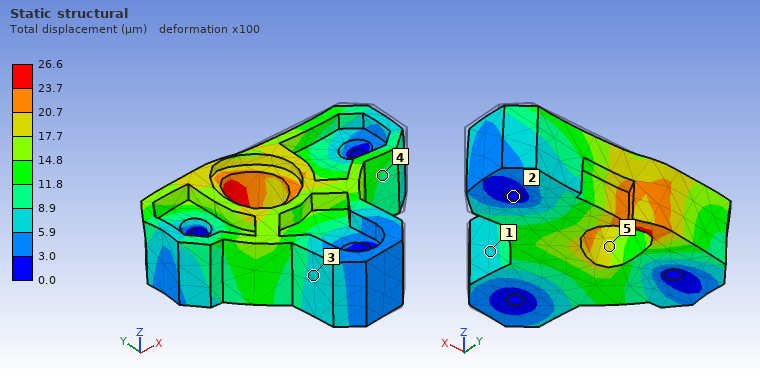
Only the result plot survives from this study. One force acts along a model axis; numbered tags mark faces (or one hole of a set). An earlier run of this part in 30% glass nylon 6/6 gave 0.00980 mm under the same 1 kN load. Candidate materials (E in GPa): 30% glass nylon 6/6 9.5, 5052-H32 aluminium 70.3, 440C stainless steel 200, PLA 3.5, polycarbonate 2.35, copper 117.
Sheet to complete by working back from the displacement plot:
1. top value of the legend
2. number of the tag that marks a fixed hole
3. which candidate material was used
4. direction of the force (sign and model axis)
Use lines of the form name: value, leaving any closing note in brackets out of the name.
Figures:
top value of the legend: 26.6 µm
number of the tag that marks a fixed hole: 2
which candidate material was used: PLA
direction of the force: -X
